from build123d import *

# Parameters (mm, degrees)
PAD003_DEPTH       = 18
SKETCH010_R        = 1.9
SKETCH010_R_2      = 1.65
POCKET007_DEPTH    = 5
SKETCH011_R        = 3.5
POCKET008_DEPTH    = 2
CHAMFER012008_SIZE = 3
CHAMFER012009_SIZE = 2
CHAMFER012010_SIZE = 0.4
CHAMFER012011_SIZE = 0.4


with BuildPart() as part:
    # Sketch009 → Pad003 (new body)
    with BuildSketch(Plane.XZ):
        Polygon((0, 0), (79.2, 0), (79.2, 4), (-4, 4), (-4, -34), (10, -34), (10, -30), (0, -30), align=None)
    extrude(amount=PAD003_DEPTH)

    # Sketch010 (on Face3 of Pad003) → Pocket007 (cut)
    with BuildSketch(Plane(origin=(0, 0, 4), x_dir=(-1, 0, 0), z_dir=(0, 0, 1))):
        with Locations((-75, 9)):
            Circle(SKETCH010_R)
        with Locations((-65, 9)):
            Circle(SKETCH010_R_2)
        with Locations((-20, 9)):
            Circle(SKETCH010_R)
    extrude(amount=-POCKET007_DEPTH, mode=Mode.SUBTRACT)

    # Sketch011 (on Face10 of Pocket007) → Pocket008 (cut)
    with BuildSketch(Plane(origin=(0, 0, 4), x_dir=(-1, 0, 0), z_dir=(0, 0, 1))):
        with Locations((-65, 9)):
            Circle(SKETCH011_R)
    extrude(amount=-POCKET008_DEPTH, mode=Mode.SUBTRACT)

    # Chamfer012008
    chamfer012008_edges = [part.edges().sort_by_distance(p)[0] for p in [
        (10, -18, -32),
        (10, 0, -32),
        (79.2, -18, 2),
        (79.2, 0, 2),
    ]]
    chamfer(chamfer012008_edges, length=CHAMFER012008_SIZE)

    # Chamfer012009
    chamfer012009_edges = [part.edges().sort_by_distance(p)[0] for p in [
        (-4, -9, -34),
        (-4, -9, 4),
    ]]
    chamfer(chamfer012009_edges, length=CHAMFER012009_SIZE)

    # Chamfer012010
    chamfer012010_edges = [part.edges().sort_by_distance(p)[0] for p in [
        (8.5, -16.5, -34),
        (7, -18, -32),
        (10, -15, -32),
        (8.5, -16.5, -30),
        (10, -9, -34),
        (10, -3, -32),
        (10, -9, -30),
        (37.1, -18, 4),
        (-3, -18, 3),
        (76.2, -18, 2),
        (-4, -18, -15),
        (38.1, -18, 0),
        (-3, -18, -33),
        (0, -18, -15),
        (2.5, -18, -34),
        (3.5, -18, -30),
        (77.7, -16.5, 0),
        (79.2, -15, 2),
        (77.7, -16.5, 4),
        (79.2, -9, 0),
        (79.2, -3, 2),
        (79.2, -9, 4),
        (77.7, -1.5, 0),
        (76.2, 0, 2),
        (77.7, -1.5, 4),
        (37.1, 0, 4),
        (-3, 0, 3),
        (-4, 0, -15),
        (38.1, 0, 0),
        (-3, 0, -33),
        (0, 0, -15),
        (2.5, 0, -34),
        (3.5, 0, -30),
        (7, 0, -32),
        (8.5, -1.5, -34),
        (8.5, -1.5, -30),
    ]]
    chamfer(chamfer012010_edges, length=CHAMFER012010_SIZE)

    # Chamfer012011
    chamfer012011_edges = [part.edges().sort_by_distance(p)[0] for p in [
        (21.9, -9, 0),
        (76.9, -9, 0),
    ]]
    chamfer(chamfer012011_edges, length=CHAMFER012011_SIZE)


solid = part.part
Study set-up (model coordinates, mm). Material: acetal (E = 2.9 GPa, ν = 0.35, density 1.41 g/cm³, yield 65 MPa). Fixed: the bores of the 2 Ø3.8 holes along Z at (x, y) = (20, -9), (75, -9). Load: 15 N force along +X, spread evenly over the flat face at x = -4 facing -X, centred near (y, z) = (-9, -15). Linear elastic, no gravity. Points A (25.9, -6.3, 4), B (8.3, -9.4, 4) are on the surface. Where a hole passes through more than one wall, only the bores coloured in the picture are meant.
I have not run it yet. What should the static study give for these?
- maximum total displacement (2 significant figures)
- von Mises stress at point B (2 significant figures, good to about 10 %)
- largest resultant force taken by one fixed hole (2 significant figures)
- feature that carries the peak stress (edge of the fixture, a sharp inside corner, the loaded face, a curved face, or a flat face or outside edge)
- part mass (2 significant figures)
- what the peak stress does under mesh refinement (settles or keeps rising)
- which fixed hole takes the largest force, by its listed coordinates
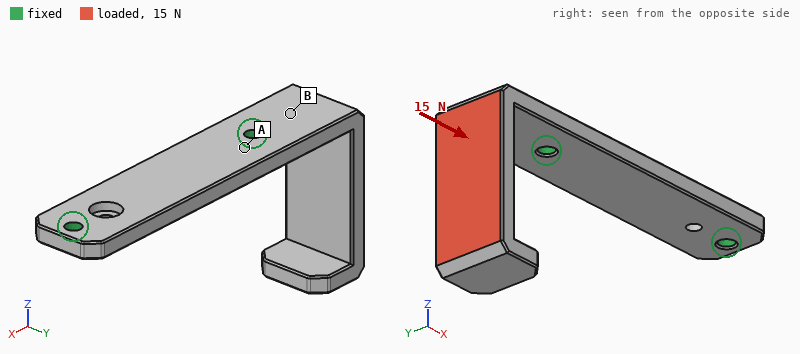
0.98 mm
4.6 MPa
14 N
edge of the fixture
12 g
keeps rising
(20, -9)
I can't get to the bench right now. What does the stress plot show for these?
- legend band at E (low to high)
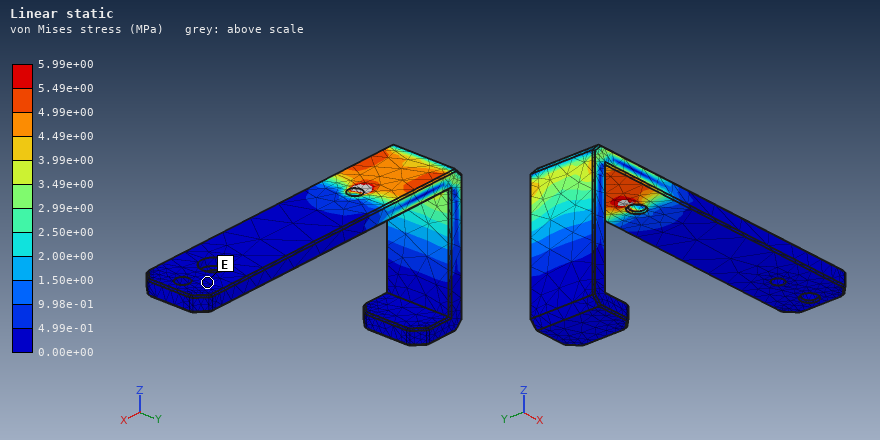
0.00e+00 to 4.99e-01 MPa
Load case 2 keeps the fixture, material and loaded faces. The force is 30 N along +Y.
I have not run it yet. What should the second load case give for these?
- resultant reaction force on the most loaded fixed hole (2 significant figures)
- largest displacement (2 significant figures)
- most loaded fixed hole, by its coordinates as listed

39 N
1.1 mm
(20, -9)
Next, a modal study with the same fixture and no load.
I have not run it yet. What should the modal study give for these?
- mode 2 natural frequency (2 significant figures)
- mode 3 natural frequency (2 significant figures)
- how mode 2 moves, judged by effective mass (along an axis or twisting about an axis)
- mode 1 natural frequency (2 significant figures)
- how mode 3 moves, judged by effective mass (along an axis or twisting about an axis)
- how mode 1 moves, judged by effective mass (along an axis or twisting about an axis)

400 Hz
880 Hz
along Y
280 Hz
along Z
along X
